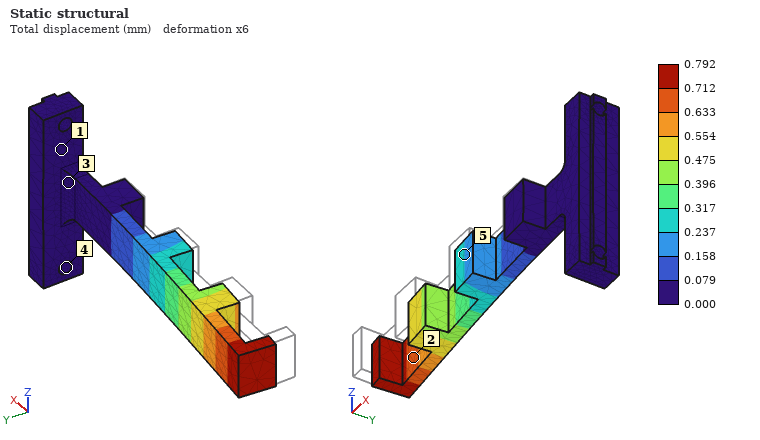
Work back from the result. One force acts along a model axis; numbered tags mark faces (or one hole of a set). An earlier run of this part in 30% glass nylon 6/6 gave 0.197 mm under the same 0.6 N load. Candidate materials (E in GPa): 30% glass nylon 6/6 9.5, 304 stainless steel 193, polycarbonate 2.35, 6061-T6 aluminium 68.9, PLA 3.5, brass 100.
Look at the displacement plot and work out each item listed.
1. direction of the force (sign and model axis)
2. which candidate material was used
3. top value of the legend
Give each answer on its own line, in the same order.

+Y
polycarbonate
0.792 mm
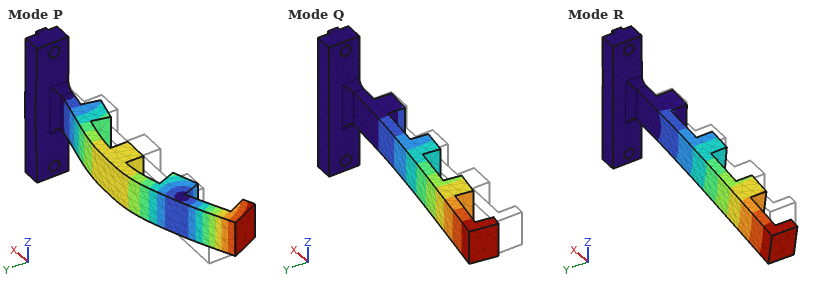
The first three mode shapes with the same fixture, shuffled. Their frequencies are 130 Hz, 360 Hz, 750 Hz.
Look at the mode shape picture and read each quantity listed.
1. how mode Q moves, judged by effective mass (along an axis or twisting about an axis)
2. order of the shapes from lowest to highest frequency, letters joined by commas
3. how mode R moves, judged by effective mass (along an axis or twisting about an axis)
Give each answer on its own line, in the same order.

along Y
Q, R, P
along Z
